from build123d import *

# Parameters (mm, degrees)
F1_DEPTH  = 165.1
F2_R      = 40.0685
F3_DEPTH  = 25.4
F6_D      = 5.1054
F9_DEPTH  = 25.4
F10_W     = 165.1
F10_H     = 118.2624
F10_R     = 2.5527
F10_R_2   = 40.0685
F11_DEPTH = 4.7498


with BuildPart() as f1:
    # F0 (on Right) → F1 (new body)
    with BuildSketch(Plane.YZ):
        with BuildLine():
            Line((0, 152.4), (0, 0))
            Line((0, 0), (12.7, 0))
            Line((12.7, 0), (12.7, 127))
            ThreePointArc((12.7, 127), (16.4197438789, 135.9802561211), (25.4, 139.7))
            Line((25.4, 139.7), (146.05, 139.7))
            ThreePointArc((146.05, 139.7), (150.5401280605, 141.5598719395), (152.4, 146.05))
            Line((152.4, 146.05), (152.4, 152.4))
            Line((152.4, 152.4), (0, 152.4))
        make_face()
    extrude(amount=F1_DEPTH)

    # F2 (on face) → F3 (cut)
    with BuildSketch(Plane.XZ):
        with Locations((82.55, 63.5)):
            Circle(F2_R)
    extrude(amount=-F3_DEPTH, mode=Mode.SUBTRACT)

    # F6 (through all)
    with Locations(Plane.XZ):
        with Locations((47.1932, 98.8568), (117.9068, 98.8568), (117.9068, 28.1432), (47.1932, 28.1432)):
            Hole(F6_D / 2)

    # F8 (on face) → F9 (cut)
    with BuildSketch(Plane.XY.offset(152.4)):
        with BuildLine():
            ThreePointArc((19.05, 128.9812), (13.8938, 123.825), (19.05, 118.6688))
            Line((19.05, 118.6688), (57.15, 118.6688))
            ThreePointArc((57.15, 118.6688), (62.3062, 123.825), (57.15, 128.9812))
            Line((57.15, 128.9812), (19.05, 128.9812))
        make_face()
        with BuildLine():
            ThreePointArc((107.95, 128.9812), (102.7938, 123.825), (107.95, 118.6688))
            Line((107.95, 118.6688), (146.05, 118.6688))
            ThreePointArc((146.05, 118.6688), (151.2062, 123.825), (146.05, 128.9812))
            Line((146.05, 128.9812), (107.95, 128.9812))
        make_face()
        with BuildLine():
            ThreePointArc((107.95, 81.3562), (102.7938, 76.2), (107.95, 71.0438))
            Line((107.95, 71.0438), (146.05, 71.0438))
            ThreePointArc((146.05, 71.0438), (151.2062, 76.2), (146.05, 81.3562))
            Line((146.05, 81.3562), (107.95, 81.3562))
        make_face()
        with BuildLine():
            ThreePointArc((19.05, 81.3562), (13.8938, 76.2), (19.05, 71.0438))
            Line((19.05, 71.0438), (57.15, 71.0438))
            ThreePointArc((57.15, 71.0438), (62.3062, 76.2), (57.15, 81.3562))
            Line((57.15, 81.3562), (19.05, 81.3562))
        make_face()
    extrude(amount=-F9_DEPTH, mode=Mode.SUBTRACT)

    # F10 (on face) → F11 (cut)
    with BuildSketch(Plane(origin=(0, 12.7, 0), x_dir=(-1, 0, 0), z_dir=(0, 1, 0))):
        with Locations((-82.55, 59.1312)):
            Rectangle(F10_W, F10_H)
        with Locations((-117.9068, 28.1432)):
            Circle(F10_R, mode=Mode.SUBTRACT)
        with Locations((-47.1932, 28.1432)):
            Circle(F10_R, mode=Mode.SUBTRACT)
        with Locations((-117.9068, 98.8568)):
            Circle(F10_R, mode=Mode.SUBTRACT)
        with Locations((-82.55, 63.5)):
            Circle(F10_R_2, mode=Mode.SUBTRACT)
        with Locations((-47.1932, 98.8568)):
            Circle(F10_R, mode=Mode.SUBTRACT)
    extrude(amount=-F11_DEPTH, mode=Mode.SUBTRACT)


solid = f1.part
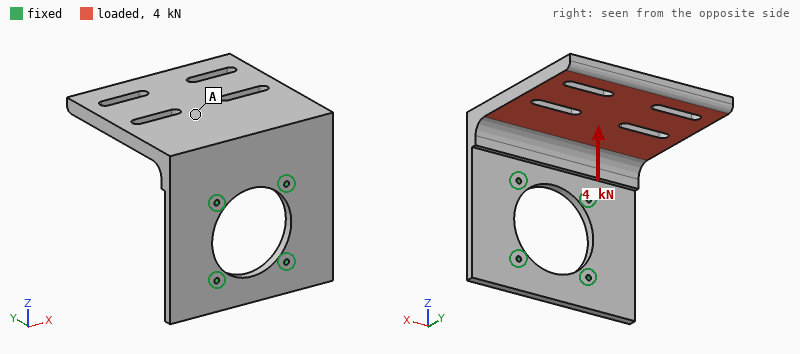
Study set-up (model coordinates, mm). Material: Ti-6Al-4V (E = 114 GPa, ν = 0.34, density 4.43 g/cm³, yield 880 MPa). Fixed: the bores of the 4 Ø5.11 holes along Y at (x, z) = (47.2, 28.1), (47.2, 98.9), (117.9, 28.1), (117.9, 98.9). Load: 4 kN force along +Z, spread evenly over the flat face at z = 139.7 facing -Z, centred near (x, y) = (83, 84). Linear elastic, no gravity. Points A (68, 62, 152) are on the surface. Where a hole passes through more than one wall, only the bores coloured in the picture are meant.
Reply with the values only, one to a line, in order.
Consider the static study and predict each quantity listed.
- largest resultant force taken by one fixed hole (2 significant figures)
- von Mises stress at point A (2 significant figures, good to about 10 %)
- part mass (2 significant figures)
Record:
2.0 kN
38 MPa
2.0 kg
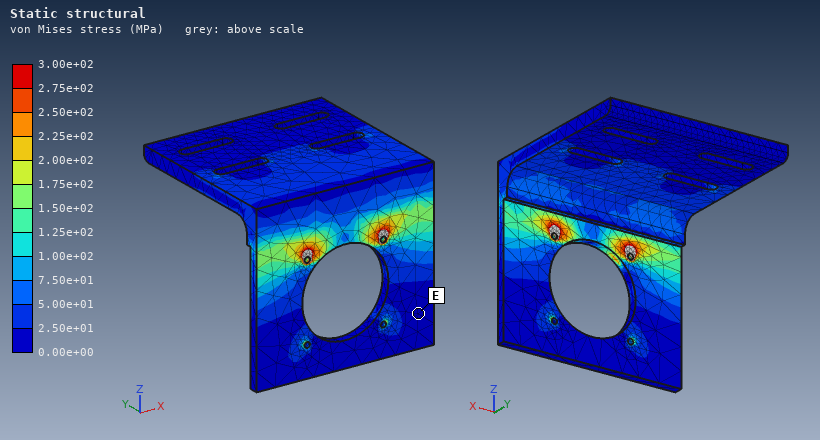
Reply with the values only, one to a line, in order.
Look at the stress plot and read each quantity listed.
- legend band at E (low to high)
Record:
0.00e+00 to 2.50e+01 MPa
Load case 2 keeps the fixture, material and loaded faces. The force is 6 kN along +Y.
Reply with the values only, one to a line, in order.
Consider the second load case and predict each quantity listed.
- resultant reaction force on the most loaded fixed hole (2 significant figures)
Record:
3.6 kN
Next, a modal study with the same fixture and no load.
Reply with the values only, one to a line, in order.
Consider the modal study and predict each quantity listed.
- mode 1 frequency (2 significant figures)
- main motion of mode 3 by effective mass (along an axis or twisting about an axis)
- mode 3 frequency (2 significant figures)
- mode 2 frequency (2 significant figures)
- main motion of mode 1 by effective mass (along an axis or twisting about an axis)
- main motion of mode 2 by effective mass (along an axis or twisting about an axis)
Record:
210 Hz
along Y
1000 Hz
520 Hz
along Z
along X
